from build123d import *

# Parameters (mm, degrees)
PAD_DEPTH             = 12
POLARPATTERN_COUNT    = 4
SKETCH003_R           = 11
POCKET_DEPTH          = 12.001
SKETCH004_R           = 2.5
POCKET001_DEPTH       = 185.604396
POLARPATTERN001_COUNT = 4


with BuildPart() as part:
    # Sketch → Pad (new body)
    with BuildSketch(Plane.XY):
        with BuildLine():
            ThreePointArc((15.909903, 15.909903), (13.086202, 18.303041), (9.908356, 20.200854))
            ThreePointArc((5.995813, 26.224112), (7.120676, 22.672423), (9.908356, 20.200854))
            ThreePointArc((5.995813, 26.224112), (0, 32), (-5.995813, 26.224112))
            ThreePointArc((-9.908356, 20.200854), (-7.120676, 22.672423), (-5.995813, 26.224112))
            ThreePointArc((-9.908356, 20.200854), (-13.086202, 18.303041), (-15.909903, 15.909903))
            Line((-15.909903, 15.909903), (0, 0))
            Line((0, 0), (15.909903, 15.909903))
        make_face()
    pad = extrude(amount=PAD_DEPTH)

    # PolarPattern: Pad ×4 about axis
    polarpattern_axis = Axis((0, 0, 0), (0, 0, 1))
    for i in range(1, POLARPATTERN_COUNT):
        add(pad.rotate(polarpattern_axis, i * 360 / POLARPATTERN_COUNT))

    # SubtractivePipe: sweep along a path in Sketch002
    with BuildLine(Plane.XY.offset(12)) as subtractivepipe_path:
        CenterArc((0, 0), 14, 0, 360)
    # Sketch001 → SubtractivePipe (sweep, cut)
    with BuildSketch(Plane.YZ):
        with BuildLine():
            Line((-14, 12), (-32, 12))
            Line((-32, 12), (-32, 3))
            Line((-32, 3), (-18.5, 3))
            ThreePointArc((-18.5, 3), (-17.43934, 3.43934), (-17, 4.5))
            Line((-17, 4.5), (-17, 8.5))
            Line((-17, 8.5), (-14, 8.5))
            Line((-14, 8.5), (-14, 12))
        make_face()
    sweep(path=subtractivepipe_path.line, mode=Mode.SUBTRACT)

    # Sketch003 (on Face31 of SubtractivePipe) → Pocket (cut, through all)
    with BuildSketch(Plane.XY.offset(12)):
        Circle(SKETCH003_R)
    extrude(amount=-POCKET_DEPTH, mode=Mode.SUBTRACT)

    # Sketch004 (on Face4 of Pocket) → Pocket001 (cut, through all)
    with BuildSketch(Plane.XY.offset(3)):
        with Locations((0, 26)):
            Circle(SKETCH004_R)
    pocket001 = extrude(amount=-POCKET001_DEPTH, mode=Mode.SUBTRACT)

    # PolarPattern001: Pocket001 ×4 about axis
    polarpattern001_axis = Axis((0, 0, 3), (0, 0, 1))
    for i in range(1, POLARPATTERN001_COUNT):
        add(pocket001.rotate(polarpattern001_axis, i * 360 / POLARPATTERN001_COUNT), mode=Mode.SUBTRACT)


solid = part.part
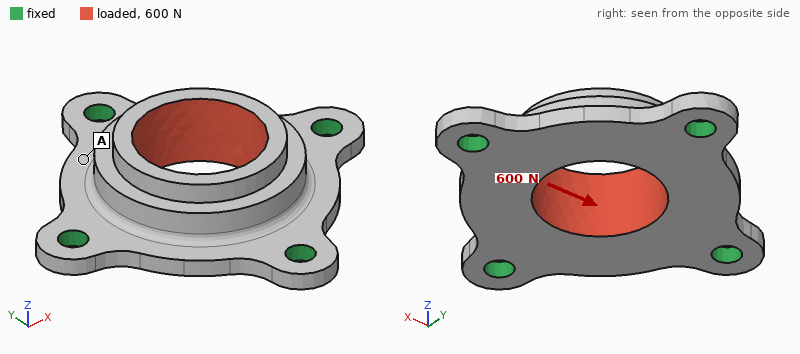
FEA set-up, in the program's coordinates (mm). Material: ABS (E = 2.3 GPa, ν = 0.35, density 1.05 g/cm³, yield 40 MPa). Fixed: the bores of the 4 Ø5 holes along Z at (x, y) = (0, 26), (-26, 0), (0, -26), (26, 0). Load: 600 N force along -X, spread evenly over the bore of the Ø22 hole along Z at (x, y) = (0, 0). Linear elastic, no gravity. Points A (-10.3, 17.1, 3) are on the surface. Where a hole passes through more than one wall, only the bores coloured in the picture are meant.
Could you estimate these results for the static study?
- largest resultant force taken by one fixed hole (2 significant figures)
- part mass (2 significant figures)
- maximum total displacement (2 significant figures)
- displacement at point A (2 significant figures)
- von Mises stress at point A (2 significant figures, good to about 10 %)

220 N
8.9 g
73 µm
39 µm
1.7 MPa
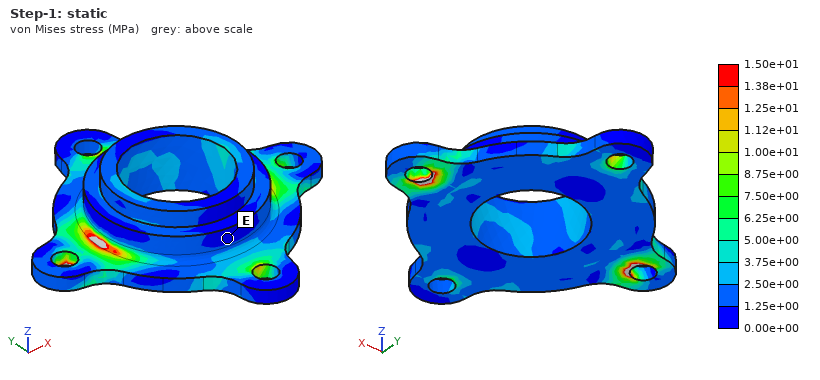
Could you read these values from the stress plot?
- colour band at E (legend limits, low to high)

0.00e+00 to 1.25e+00 MPa
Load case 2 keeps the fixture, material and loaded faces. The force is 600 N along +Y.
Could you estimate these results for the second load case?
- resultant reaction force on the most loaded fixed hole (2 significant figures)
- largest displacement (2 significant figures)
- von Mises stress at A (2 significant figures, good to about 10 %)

220 N
74 µm
3.8 MPa
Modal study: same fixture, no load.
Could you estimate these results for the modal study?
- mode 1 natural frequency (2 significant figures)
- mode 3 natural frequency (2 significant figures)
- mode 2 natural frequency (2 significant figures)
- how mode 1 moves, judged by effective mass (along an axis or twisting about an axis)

3500 Hz
4500 Hz
4500 Hz
along Z
